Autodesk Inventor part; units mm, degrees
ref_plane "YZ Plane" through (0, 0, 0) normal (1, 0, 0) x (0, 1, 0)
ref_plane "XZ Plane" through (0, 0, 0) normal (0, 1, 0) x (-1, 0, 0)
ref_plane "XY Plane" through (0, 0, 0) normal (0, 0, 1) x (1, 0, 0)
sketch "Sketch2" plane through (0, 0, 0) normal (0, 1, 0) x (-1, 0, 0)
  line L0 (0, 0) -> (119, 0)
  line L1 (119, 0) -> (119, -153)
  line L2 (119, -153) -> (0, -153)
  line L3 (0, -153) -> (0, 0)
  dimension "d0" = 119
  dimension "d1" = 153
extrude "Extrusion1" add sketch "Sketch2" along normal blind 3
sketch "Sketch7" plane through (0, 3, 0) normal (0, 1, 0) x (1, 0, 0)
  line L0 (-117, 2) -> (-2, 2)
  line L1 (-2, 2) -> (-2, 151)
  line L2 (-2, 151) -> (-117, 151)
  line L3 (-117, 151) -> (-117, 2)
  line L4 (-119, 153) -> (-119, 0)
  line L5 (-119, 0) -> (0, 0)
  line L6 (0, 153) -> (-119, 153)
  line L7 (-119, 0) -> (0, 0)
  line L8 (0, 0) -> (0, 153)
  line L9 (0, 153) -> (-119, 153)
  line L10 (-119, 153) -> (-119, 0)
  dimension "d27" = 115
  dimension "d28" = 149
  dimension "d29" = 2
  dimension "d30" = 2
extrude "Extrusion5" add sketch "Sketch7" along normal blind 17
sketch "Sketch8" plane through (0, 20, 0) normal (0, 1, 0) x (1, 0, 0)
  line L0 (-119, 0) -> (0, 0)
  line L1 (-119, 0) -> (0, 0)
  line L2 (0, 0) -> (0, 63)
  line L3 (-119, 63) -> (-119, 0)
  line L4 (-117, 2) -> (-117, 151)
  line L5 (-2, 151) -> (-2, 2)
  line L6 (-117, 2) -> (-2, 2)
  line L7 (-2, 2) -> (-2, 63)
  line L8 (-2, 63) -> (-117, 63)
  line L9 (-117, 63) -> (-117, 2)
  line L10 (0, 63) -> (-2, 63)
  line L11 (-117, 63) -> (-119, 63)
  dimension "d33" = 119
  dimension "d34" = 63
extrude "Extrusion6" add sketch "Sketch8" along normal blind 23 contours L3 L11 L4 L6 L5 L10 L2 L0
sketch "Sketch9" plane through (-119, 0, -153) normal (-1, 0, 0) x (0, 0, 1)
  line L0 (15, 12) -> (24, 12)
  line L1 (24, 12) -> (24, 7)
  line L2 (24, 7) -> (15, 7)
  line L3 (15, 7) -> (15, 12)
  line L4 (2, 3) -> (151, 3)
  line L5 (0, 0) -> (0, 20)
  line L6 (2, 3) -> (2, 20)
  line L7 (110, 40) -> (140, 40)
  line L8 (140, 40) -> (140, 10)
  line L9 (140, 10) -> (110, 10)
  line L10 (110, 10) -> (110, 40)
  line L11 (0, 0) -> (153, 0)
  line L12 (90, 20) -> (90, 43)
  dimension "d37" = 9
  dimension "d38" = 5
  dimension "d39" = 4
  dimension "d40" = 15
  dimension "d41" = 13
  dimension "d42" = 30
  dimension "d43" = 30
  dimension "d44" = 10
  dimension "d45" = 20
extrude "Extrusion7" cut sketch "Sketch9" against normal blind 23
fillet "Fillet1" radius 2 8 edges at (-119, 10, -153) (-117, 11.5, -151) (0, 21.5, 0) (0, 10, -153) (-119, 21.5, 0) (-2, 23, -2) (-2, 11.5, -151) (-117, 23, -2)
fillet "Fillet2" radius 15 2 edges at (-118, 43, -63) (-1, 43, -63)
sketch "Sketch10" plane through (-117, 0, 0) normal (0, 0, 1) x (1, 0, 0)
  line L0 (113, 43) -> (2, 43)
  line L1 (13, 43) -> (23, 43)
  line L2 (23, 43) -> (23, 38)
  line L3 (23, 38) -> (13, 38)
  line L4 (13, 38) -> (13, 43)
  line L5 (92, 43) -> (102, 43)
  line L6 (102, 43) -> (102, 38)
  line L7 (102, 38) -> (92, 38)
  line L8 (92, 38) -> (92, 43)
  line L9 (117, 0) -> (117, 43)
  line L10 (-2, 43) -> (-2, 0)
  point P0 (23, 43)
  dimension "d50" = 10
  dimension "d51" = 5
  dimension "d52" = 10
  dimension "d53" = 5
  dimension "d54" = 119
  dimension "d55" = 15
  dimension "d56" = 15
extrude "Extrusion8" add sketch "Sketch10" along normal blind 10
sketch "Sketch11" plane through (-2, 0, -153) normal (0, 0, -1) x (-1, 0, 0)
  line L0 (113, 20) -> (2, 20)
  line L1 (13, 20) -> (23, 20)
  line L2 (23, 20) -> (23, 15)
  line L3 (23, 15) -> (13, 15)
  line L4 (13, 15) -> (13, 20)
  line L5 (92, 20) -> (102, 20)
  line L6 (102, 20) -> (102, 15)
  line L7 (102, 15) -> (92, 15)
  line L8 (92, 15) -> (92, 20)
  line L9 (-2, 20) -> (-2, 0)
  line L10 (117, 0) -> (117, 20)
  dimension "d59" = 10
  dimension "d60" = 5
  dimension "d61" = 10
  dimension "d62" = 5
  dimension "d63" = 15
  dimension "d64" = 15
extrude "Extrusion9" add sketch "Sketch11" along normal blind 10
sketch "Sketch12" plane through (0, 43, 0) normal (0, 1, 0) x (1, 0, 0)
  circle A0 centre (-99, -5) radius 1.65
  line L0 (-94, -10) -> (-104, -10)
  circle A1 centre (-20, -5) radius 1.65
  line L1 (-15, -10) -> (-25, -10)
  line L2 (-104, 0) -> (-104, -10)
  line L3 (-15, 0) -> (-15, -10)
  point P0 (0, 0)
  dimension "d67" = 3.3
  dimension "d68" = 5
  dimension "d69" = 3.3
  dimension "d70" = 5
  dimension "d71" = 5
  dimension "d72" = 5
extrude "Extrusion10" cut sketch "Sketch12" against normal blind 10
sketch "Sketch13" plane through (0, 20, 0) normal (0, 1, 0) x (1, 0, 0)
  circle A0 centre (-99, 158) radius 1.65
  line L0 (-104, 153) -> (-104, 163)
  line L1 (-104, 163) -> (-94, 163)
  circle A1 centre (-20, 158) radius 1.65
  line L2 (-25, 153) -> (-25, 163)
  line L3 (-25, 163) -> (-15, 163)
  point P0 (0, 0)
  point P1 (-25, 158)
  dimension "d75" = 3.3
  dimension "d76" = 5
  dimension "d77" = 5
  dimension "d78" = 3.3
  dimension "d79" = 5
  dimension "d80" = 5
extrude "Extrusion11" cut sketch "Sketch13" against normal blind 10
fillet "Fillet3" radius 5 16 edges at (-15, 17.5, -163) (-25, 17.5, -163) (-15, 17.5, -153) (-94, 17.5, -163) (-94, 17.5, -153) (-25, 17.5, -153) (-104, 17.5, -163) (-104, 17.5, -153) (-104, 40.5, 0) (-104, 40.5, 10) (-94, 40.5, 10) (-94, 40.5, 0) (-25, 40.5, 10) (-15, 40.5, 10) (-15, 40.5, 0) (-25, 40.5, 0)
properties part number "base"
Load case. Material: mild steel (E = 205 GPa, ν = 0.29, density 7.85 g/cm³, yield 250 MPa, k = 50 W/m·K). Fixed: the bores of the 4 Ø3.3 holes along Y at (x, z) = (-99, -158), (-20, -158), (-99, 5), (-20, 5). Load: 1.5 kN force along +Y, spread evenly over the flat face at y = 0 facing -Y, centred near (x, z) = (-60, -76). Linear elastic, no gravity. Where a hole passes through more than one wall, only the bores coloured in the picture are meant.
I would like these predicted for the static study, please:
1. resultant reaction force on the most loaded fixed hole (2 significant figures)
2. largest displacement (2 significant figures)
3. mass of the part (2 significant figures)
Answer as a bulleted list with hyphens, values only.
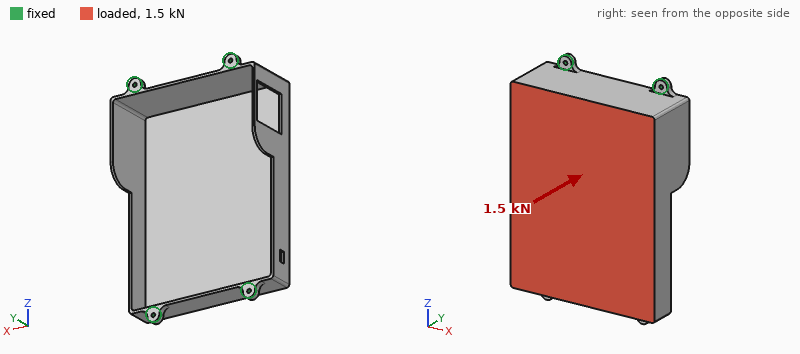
- 430 N
- 0.17 mm
- 660 g
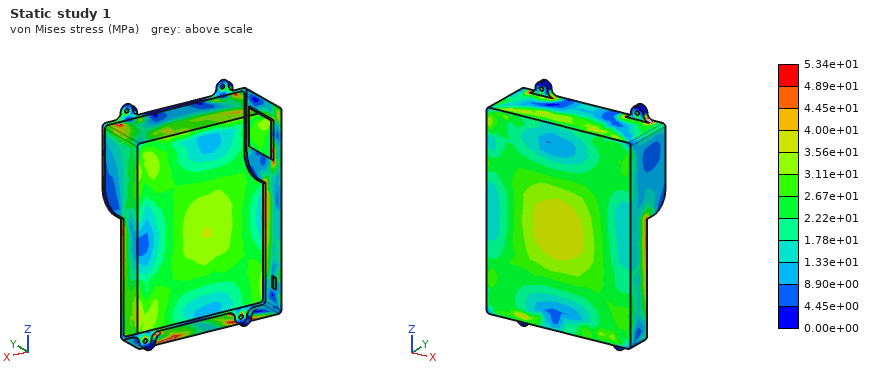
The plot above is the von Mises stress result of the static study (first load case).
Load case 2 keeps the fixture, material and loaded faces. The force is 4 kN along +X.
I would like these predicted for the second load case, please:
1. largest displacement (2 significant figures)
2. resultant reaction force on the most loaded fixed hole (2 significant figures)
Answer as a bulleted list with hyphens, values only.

- 20 µm
- 1.4 kN
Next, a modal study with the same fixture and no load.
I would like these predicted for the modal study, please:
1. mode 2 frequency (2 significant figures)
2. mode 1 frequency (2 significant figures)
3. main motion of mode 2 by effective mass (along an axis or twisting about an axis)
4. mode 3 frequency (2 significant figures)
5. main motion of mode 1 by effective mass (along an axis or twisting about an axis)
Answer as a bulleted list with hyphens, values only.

- 1300 Hz
- 860 Hz
- along Z
- 1500 Hz
- along Y
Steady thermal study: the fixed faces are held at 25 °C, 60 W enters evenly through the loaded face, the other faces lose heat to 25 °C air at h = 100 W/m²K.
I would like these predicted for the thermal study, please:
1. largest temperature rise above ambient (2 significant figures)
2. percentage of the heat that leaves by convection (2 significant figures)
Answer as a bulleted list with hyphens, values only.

- 24 K
- 93 %
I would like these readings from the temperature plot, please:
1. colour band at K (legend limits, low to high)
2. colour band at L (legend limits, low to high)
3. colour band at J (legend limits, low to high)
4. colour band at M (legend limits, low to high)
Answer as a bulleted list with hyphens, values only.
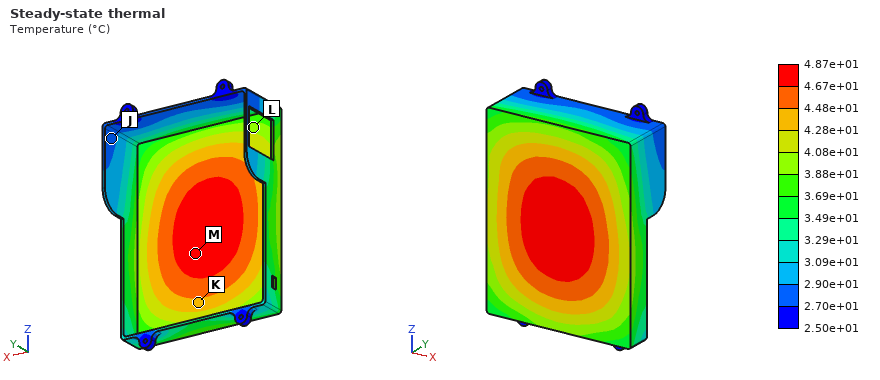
- 4.28e+01 to 4.48e+01 °C
- 3.88e+01 to 4.08e+01 °C
- 2.70e+01 to 2.90e+01 °C
- 4.67e+01 to 4.87e+01 °C
